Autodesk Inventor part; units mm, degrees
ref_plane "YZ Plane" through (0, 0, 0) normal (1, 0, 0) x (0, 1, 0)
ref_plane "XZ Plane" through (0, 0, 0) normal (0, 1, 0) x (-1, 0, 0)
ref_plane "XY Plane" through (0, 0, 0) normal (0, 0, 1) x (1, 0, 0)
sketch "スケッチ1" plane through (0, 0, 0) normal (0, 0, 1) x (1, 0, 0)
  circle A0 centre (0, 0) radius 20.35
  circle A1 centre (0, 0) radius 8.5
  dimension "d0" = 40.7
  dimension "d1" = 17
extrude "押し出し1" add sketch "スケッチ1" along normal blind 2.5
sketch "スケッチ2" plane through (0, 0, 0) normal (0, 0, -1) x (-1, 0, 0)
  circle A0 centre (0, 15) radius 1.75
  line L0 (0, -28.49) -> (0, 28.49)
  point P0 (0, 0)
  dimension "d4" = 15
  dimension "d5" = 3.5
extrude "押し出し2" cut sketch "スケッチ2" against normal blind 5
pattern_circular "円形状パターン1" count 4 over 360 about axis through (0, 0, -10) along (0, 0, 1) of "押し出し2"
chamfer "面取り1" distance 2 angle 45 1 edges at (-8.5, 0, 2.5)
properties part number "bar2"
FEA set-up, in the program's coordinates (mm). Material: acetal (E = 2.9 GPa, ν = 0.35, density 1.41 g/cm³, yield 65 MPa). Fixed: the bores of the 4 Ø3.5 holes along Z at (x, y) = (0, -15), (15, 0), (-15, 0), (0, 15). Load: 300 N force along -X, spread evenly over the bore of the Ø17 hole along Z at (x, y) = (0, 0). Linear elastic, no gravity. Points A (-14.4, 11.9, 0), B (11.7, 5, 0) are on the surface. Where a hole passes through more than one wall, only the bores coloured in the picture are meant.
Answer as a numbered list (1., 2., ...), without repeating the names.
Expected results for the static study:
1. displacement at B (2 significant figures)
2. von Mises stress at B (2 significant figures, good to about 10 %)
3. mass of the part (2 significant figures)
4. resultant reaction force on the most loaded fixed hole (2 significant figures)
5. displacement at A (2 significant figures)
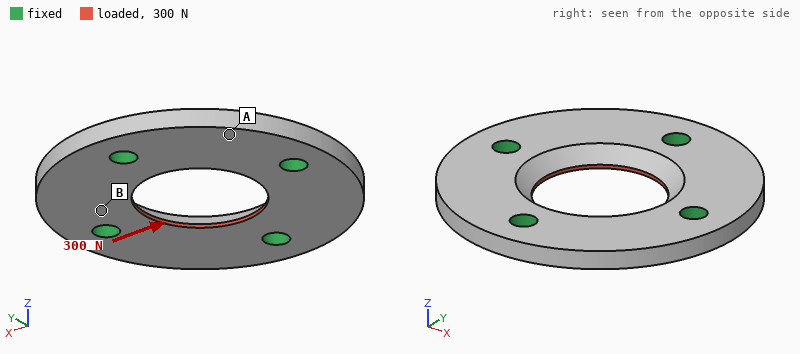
1. 9.9 µm
2. 4.3 MPa
3. 3.5 g
4. 77 N
5. 15 µm
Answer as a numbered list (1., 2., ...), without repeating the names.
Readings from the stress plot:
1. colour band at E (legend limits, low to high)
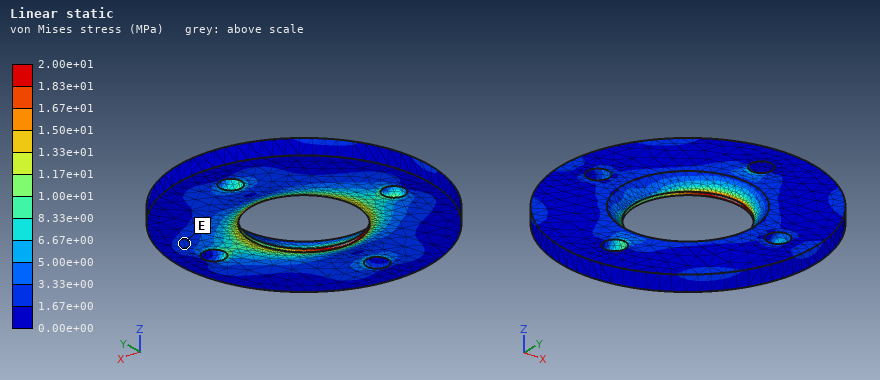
1. 1.67e+00 to 3.33e+00 MPa
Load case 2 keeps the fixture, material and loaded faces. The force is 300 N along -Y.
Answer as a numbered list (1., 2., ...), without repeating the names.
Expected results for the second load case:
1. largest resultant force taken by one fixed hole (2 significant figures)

1. 77 N
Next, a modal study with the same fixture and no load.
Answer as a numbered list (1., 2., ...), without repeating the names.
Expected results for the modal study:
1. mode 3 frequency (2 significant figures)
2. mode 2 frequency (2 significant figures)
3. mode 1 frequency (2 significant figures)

1. 5700 Hz
2. 5700 Hz
3. 5500 Hz
